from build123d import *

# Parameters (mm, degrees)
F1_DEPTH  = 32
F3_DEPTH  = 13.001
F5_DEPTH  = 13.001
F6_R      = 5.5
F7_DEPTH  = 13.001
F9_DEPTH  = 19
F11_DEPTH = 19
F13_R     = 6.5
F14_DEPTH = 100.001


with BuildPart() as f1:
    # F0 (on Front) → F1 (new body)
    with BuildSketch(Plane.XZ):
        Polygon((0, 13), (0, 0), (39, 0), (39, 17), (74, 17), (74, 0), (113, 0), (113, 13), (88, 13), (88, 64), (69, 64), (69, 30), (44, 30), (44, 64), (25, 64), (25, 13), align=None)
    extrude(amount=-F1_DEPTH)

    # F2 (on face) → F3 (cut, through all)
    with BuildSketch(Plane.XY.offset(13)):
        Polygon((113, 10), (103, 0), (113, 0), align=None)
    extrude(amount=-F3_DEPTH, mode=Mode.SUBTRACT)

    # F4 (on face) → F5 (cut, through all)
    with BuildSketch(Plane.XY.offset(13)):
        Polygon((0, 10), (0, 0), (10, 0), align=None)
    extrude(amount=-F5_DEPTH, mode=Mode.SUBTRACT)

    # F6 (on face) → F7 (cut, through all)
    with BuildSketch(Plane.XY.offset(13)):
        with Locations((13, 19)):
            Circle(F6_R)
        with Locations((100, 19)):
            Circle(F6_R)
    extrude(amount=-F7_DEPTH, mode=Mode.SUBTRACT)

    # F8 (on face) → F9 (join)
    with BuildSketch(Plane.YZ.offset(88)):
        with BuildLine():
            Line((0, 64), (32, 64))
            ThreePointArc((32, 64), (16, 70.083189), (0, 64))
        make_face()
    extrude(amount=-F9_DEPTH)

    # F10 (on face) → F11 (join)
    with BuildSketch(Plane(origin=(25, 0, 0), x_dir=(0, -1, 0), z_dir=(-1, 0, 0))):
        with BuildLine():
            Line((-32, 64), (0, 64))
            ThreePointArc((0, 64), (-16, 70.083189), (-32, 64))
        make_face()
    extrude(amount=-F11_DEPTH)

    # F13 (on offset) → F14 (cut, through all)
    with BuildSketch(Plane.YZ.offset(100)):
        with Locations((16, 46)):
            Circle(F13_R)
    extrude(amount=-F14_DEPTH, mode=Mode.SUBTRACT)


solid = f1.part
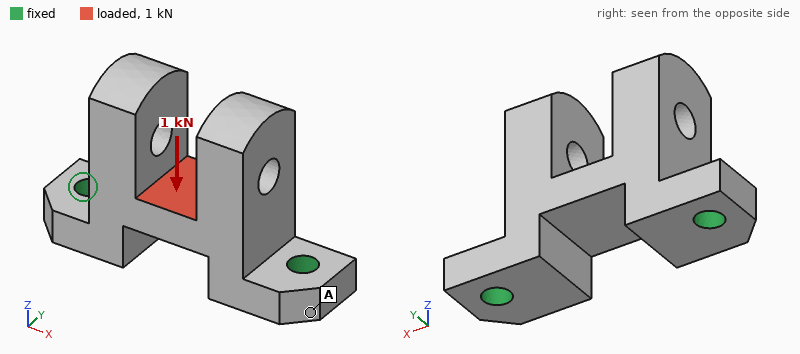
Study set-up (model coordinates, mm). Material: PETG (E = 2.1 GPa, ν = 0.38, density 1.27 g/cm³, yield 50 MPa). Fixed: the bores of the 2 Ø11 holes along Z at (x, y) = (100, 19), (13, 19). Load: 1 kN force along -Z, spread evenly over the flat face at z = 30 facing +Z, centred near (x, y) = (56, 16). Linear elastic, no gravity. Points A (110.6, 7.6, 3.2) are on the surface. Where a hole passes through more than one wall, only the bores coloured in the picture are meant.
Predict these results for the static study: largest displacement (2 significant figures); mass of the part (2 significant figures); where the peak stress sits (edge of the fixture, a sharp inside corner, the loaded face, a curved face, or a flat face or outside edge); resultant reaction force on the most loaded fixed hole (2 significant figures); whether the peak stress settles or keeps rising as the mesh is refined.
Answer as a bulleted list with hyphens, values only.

- 0.18 mm
- 130 g
- edge of the fixture
- 740 N
- keeps rising
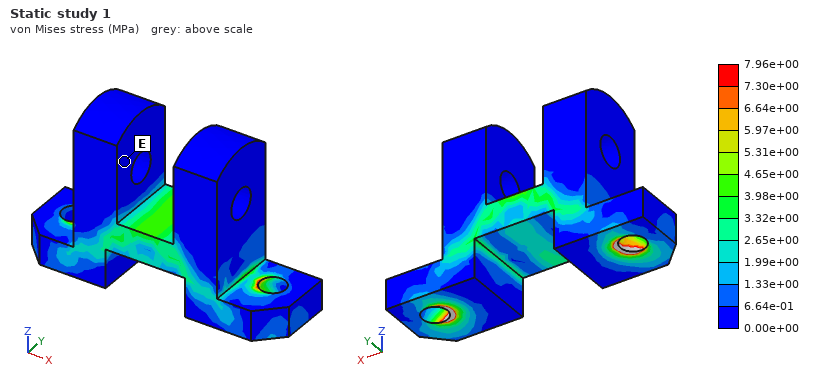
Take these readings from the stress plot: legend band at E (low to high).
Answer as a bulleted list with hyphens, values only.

- 0.00e+00 to 6.64e-01 MPa
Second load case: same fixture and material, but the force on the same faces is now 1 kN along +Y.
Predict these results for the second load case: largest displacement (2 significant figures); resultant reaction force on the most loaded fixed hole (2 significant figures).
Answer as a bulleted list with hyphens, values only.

- 0.78 mm
- 500 N
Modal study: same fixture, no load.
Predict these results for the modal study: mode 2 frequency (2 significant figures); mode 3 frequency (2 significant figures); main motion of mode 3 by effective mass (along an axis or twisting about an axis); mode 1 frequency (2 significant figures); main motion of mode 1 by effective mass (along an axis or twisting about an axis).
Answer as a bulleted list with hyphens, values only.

- 1000 Hz
- 1200 Hz
- along X
- 610 Hz
- along Y
